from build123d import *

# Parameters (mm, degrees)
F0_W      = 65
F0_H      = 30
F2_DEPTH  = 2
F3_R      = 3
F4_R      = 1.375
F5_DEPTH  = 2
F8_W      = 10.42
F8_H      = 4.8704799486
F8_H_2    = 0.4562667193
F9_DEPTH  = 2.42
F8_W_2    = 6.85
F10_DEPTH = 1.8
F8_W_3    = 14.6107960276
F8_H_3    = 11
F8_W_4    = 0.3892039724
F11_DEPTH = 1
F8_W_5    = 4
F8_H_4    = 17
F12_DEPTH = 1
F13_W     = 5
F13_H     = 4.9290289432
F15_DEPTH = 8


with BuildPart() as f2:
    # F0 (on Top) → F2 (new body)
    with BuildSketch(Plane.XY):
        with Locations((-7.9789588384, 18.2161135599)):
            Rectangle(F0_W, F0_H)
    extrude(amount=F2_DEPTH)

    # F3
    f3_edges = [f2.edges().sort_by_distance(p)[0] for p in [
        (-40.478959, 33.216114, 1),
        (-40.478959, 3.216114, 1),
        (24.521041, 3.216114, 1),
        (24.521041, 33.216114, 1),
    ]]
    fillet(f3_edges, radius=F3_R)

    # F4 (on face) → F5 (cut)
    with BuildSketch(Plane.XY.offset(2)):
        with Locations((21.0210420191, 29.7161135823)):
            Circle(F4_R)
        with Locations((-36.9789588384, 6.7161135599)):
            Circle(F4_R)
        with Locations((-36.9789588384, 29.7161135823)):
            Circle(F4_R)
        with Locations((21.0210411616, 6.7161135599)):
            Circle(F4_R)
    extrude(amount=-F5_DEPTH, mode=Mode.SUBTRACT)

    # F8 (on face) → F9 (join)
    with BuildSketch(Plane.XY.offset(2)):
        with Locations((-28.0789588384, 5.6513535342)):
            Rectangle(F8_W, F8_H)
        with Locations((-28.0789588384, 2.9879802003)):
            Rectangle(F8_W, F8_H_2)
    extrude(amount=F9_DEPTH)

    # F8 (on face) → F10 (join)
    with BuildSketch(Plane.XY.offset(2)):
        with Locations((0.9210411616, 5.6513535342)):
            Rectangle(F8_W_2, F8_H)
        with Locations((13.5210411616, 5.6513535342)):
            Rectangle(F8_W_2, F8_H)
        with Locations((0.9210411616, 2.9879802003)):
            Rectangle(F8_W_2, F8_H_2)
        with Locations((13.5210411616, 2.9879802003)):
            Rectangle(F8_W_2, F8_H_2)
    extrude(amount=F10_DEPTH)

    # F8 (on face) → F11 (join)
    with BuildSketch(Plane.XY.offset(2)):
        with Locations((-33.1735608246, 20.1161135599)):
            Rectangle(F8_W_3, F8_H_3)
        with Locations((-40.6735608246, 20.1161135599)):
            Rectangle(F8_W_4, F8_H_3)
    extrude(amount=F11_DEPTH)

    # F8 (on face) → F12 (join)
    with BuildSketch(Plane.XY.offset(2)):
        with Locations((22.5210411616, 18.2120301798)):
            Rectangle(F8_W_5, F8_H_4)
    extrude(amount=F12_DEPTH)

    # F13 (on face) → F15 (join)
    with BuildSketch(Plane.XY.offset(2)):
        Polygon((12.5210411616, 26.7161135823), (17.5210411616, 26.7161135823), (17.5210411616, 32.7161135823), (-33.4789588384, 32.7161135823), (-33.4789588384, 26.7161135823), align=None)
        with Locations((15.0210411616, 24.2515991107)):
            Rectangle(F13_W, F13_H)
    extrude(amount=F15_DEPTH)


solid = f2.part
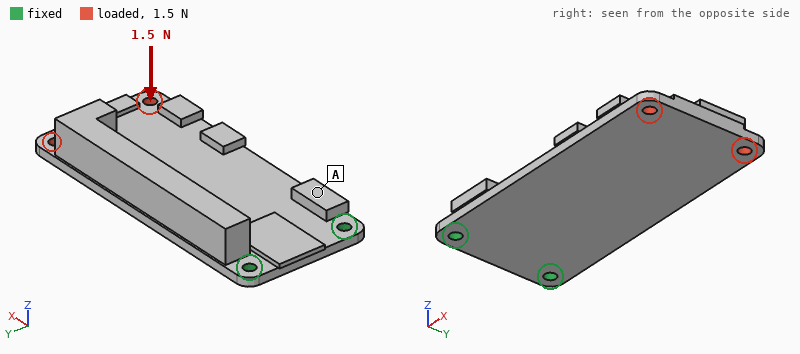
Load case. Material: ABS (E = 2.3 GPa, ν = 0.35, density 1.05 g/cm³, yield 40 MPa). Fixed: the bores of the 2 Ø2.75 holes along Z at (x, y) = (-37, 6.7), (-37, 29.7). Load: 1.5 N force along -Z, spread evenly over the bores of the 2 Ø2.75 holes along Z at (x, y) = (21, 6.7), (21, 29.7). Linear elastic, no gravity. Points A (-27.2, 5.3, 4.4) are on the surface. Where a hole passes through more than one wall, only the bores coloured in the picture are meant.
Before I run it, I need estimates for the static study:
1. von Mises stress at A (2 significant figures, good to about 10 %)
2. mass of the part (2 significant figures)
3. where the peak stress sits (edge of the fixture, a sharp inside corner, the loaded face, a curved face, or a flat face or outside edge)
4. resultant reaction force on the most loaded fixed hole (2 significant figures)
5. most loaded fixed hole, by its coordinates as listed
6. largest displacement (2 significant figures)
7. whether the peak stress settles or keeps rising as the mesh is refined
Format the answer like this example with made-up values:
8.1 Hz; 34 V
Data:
0.73 MPa; 7.3 g; edge of the fixture; 1.6 N; (-37, 6.7); 0.73 mm; keeps rising
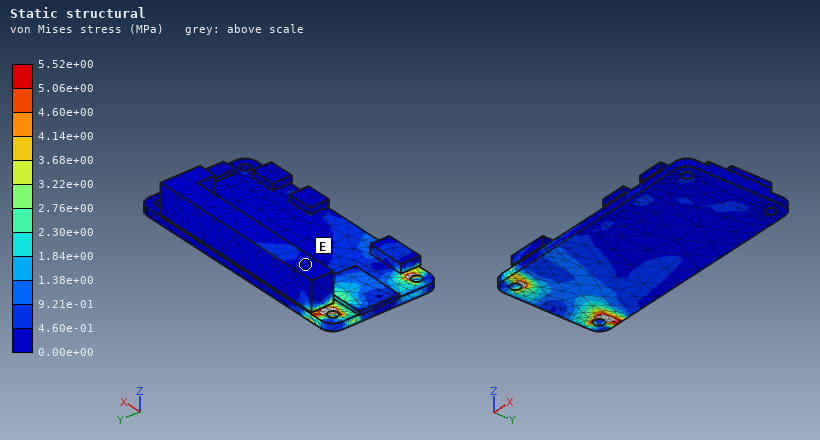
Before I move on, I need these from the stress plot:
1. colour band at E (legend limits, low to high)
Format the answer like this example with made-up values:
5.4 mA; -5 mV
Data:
0.00e+00 to 4.60e-01 MPa
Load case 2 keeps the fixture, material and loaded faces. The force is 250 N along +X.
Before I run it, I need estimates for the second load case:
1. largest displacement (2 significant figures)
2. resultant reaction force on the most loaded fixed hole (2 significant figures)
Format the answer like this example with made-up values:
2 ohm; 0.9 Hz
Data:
0.50 mm; 130 N
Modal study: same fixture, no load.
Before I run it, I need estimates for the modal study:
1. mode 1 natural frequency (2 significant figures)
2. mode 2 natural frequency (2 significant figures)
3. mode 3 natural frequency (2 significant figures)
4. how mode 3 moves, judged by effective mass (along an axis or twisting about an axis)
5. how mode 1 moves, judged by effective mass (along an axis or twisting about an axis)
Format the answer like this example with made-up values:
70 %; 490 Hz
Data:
160 Hz; 700 Hz; 1300 Hz; along Y; along Z
